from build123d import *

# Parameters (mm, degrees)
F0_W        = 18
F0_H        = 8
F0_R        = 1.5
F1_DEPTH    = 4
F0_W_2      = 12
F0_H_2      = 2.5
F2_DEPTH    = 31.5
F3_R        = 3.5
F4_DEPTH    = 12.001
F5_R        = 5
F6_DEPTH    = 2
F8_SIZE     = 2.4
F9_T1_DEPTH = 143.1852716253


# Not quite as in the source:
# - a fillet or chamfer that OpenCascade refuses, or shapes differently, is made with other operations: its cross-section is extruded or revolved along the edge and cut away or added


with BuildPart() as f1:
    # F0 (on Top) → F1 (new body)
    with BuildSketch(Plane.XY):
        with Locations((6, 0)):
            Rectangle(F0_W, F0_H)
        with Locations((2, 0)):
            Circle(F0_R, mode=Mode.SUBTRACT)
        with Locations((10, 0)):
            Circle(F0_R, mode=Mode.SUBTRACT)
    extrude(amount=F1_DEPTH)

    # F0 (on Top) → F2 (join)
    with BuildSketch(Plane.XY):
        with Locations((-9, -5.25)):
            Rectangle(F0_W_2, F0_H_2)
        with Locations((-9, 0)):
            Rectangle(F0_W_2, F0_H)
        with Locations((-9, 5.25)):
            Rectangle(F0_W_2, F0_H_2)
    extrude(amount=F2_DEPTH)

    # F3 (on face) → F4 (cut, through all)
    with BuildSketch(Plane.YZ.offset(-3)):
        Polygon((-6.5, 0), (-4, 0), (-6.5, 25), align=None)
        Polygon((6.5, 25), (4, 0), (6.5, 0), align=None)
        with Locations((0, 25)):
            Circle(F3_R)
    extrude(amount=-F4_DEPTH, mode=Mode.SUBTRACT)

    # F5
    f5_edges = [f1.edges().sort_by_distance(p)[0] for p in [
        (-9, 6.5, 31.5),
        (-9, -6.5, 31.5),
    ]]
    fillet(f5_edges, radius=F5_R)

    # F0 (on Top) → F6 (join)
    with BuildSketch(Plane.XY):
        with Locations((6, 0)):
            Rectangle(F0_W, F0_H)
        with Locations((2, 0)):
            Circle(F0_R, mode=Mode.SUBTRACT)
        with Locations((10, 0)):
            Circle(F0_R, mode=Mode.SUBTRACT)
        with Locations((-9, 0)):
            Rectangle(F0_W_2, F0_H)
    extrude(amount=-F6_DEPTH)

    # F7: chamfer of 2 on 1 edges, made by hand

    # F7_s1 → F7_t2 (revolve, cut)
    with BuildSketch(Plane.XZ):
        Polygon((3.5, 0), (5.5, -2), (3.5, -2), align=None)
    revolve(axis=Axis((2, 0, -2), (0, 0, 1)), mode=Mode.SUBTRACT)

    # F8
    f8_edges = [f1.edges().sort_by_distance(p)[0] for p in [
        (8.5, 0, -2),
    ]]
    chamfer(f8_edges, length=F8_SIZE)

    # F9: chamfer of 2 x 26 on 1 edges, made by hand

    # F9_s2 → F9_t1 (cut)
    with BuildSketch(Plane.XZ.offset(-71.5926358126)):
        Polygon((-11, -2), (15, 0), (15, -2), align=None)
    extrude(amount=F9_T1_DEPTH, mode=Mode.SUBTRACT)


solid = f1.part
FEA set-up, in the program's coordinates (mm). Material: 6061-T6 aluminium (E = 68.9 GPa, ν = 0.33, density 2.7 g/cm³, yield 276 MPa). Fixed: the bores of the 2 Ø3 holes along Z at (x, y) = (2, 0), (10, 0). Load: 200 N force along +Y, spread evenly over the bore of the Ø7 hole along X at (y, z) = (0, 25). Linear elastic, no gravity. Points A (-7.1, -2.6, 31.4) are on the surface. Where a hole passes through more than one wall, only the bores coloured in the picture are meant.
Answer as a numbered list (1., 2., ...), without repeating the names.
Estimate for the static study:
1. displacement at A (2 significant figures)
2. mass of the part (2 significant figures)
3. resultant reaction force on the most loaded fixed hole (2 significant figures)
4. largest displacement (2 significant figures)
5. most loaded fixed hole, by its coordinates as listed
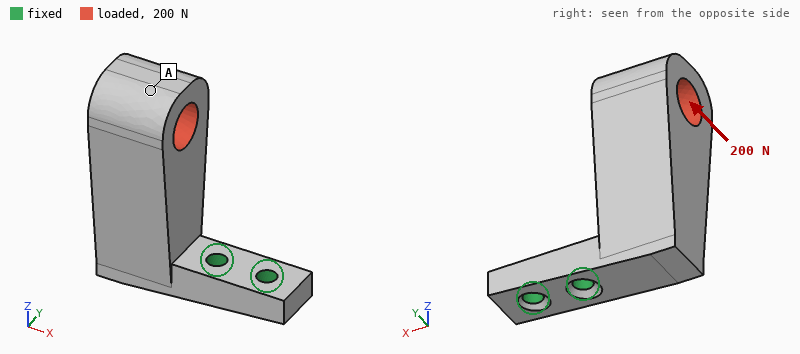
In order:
1. 0.18 mm
2. 12 g
3. 310 N
4. 0.19 mm
5. (2, 0)
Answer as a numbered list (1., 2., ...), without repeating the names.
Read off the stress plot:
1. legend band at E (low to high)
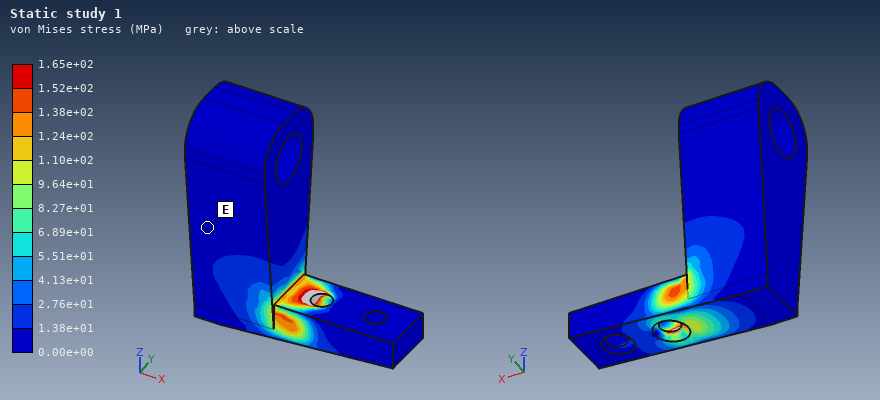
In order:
1. 0.00e+00 to 1.38e+01 MPa
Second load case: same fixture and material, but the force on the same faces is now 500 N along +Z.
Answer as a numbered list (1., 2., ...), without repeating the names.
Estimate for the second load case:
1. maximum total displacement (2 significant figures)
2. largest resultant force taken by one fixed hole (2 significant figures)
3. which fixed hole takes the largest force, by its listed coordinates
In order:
1. 0.16 mm
2. 630 N
3. (2, 0)
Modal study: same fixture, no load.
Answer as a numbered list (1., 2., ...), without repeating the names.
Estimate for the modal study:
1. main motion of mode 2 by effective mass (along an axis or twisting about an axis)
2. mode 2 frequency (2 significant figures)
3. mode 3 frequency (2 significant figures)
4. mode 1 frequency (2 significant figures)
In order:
1. along Y
2. 2600 Hz
3. 8800 Hz
4. 2500 Hz
